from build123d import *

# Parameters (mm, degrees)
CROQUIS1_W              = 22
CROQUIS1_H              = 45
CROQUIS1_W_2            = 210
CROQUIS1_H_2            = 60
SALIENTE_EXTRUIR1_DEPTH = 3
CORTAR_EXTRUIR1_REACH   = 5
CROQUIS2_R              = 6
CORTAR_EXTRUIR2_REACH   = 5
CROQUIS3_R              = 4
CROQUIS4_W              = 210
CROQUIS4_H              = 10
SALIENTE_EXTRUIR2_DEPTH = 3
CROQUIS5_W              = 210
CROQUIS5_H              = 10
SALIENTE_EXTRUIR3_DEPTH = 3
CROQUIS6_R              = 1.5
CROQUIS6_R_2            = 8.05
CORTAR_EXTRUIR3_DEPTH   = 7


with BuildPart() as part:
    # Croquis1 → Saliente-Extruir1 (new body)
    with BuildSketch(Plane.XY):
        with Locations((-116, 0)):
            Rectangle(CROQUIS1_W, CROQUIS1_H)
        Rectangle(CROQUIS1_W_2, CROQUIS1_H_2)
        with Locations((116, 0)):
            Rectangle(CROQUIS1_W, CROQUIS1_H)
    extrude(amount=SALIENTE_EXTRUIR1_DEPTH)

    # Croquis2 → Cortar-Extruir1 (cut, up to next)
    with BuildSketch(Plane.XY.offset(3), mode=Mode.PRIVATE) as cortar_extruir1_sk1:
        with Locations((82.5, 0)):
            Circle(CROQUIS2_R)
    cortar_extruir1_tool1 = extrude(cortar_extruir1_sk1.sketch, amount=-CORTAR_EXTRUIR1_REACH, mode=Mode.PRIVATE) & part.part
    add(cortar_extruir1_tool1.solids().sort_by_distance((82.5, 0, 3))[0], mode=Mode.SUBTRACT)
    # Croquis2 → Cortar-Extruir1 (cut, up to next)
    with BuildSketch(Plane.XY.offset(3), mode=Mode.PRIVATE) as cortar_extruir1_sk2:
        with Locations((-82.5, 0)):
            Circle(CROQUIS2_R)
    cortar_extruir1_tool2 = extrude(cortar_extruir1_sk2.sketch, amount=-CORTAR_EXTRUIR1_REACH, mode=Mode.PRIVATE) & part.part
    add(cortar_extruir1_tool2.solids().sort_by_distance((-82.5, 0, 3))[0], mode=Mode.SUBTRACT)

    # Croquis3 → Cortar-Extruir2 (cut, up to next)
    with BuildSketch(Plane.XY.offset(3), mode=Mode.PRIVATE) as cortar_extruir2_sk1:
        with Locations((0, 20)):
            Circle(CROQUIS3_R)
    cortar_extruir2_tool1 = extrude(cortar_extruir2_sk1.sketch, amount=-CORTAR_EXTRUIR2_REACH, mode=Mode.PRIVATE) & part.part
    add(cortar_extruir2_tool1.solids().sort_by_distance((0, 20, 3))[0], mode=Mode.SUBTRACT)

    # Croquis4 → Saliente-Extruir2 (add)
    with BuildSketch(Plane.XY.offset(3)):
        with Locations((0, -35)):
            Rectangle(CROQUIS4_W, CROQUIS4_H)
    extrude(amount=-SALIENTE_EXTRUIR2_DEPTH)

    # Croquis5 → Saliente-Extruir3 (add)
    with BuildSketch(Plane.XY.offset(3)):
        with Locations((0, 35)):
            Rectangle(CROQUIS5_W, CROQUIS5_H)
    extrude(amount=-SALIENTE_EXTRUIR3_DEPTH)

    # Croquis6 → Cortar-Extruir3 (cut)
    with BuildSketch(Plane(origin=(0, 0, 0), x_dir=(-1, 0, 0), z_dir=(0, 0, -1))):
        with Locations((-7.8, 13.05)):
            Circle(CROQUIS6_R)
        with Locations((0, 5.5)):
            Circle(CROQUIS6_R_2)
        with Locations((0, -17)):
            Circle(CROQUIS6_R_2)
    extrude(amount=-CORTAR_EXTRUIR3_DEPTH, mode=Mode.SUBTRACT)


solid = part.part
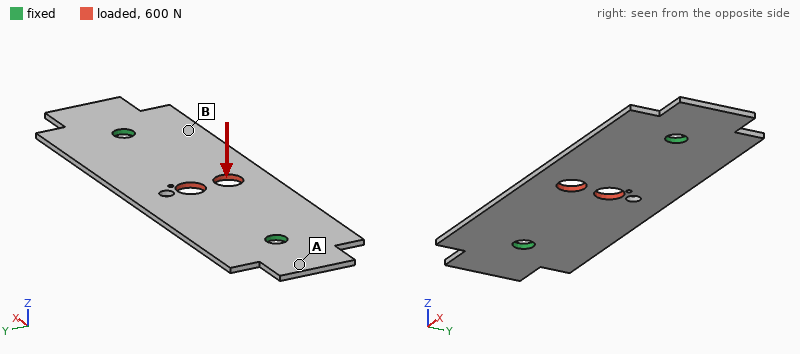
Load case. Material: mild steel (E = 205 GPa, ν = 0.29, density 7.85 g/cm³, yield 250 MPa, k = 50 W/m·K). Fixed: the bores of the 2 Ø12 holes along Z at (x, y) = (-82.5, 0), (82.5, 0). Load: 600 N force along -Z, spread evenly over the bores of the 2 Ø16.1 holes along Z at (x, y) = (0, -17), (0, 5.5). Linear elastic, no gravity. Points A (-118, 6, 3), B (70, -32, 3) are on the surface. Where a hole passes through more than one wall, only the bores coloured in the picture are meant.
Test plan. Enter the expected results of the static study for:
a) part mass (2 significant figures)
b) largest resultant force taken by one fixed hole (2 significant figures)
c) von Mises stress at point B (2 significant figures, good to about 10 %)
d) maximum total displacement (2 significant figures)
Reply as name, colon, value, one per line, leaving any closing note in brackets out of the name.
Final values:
part mass: 430 g
largest resultant force taken by one fixed hole: 300 N
von Mises stress at point B: 58 MPa
maximum total displacement: 0.51 mm
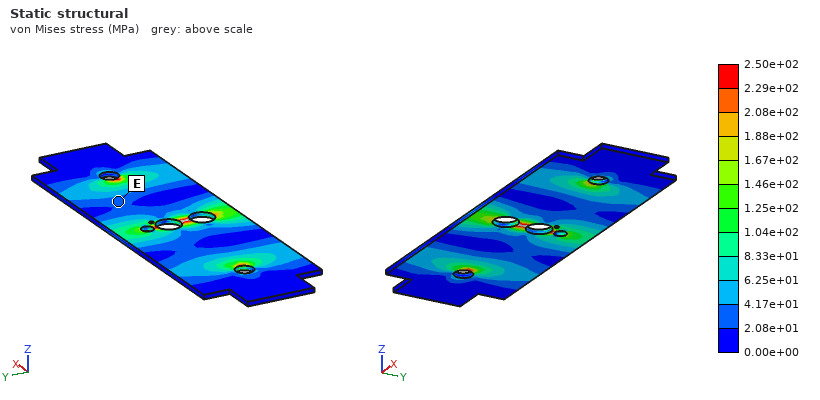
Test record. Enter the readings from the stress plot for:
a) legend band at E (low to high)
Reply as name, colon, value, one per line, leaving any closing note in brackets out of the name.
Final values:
legend band at E: 2.08e+01 to 4.17e+01 MPa
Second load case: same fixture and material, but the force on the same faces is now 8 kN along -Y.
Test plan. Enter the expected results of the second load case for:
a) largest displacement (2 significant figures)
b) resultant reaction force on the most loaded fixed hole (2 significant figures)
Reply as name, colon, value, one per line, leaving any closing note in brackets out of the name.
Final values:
largest displacement: 49 µm
resultant reaction force on the most loaded fixed hole: 4.0 kN
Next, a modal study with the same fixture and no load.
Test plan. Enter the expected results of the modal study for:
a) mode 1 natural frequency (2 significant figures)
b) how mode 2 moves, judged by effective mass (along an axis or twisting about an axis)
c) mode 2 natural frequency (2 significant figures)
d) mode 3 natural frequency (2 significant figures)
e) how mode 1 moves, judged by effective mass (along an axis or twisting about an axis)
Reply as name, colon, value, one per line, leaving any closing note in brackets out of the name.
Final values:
mode 1 natural frequency: 560 Hz
how mode 2 moves, judged by effective mass: twisting about X
mode 2 natural frequency: 760 Hz
mode 3 natural frequency: 1400 Hz
how mode 1 moves, judged by effective mass: along Z
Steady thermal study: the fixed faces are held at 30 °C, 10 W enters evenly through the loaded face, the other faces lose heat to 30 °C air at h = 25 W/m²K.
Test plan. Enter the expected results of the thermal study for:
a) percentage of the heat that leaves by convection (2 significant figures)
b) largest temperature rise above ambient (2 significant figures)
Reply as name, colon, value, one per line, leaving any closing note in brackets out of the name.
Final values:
percentage of the heat that leaves by convection: 65 %
largest temperature rise above ambient: 28 K
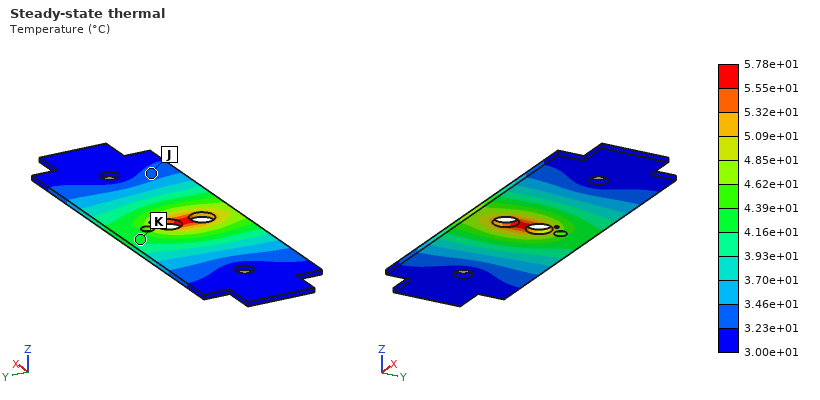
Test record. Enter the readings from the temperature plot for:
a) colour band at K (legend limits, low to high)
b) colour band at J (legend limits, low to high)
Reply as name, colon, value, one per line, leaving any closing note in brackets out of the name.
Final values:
colour band at K: 4.16e+01 to 4.39e+01 °C
colour band at J: 3.23e+01 to 3.46e+01 °C
